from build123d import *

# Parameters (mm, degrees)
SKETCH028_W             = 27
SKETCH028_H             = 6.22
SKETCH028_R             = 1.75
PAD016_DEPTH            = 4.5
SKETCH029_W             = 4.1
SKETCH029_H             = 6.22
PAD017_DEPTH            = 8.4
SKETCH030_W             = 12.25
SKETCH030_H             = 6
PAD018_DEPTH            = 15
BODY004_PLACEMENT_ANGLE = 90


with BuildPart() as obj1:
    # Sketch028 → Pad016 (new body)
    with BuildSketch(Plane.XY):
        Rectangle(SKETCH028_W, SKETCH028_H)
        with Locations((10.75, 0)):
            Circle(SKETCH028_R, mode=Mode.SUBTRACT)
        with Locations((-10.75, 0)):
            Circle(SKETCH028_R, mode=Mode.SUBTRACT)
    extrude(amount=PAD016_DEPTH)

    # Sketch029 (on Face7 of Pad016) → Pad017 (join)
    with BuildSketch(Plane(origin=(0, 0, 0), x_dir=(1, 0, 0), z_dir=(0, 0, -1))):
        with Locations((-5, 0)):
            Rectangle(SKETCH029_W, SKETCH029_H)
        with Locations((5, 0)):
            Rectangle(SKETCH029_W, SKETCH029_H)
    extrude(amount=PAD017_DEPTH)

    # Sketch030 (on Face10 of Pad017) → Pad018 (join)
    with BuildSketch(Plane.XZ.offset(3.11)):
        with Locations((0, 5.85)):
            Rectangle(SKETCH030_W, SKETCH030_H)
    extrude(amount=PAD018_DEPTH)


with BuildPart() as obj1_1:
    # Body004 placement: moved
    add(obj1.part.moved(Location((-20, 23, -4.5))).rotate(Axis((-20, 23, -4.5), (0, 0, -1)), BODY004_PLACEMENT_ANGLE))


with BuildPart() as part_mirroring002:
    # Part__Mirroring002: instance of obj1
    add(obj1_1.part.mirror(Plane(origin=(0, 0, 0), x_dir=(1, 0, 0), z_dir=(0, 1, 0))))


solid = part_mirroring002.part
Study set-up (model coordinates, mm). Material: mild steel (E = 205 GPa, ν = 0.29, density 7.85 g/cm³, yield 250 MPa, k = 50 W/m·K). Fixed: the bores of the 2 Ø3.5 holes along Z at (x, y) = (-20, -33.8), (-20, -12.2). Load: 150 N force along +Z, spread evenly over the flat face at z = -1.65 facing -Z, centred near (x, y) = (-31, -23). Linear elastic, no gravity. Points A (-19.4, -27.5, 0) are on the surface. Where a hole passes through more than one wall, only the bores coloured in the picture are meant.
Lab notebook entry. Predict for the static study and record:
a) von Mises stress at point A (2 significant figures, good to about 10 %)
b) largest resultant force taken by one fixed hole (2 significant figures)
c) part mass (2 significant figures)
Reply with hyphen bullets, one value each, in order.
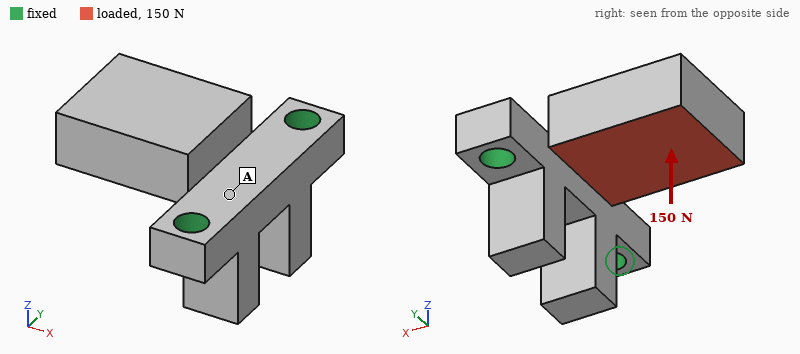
- 23 MPa
- 75 N
- 17 g
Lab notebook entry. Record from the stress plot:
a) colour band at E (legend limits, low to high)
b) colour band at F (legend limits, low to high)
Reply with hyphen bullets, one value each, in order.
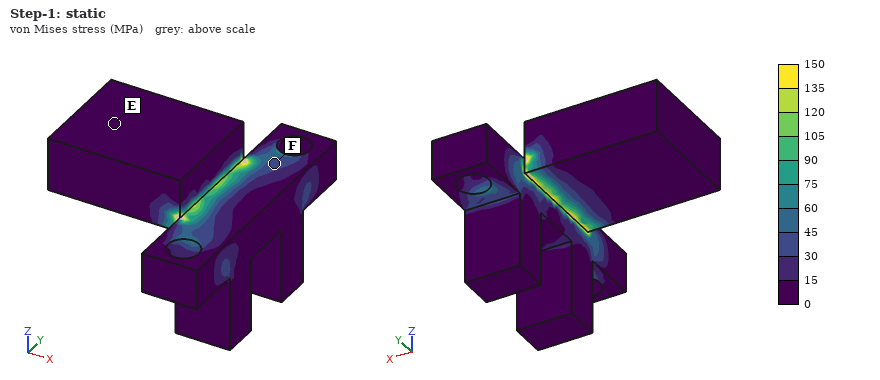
- 0 to 15 MPa
- 30 to 45 MPa
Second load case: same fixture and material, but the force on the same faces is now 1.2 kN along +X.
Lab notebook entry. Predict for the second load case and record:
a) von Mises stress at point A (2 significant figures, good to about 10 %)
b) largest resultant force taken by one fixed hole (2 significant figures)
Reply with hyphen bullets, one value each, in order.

- 38 MPa
- 620 N
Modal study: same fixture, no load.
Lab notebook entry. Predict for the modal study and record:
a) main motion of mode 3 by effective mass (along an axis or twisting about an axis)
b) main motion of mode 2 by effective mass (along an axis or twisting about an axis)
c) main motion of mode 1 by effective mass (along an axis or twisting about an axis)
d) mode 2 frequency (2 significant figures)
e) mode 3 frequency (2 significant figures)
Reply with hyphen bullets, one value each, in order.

- along X
- along Y
- along Z
- 15 kHz
- 22 kHz
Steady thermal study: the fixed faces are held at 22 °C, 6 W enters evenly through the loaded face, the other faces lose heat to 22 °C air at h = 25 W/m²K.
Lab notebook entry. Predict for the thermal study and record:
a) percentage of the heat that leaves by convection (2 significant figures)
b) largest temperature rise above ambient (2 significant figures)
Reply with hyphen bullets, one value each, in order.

- 8.2 %
- 34 K
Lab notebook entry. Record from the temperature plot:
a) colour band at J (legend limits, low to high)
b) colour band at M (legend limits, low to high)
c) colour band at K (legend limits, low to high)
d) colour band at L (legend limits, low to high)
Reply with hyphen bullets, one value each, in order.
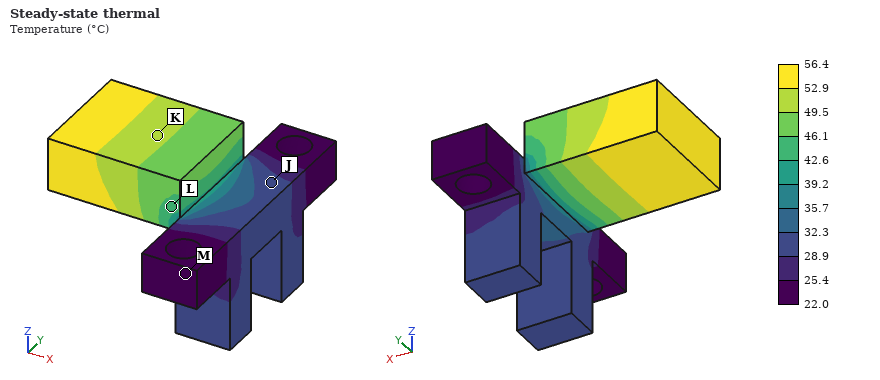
- 28.9 to 32.3 °C
- 22.0 to 25.4 °C
- 49.5 to 52.9 °C
- 42.6 to 46.1 °C
